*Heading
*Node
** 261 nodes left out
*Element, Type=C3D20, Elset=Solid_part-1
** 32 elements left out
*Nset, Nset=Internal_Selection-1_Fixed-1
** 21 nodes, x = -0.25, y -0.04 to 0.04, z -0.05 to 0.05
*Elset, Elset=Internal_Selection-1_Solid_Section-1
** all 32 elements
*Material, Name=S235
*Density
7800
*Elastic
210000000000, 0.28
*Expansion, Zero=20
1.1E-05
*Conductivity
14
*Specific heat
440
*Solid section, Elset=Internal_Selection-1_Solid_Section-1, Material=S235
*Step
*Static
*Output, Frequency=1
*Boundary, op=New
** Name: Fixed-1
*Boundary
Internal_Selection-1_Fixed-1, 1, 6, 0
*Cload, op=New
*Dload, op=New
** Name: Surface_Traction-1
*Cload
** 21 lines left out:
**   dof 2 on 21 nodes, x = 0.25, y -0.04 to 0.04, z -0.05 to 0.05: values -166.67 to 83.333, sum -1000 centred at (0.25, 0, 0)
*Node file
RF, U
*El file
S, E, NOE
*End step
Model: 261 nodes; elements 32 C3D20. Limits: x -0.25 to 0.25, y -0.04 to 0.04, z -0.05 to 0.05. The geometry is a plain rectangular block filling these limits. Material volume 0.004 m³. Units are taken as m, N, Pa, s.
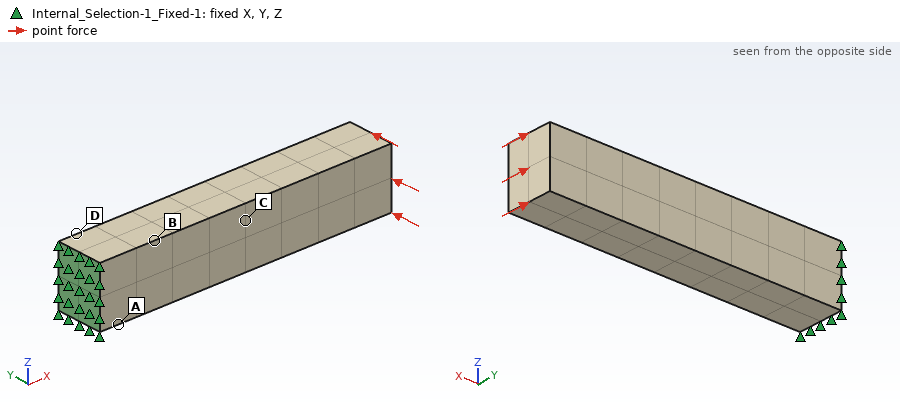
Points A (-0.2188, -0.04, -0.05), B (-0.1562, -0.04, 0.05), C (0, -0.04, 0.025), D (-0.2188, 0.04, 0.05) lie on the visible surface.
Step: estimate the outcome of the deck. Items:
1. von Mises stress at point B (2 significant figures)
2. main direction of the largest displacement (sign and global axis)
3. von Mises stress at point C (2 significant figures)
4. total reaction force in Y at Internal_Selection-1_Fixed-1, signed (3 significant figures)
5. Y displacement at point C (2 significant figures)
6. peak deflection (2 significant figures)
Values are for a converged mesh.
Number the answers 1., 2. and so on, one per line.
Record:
1. 3.8e+06 Pa
2. -Y
3. 2.3e+06 Pa
4. 1000 N
5. -1.5e-05 m
6. 4.7e-05 m
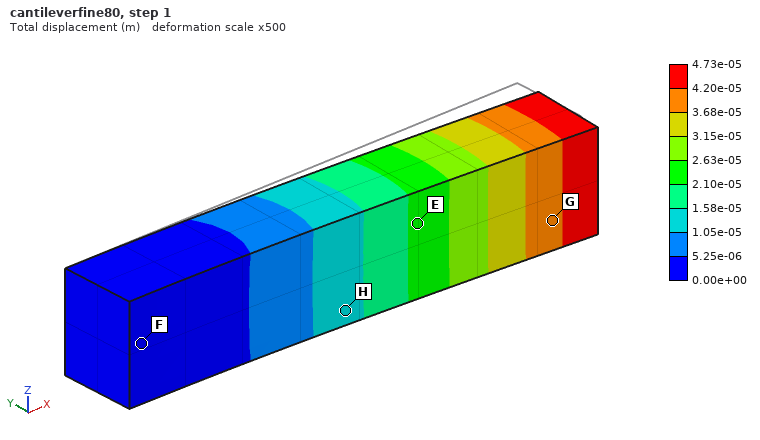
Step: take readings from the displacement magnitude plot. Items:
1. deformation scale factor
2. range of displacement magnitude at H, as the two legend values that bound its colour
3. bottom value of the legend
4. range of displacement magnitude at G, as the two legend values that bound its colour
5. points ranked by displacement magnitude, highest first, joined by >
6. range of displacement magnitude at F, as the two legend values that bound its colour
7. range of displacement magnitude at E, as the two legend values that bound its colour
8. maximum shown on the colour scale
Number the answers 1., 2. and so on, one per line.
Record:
1. 500
2. 1.05e-05 to 1.58e-05 m
3. 0.00e+00 m
4. 3.68e-05 to 4.20e-05 m
5. G > E > H > F
6. 0.00e+00 to 5.25e-06 m
7. 2.10e-05 to 2.63e-05 m
8. 4.73e-05 m
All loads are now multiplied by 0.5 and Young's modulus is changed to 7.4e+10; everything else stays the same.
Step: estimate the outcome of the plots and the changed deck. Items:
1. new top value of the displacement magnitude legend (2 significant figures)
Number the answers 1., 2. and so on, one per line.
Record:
1. 6.7e-05 m
